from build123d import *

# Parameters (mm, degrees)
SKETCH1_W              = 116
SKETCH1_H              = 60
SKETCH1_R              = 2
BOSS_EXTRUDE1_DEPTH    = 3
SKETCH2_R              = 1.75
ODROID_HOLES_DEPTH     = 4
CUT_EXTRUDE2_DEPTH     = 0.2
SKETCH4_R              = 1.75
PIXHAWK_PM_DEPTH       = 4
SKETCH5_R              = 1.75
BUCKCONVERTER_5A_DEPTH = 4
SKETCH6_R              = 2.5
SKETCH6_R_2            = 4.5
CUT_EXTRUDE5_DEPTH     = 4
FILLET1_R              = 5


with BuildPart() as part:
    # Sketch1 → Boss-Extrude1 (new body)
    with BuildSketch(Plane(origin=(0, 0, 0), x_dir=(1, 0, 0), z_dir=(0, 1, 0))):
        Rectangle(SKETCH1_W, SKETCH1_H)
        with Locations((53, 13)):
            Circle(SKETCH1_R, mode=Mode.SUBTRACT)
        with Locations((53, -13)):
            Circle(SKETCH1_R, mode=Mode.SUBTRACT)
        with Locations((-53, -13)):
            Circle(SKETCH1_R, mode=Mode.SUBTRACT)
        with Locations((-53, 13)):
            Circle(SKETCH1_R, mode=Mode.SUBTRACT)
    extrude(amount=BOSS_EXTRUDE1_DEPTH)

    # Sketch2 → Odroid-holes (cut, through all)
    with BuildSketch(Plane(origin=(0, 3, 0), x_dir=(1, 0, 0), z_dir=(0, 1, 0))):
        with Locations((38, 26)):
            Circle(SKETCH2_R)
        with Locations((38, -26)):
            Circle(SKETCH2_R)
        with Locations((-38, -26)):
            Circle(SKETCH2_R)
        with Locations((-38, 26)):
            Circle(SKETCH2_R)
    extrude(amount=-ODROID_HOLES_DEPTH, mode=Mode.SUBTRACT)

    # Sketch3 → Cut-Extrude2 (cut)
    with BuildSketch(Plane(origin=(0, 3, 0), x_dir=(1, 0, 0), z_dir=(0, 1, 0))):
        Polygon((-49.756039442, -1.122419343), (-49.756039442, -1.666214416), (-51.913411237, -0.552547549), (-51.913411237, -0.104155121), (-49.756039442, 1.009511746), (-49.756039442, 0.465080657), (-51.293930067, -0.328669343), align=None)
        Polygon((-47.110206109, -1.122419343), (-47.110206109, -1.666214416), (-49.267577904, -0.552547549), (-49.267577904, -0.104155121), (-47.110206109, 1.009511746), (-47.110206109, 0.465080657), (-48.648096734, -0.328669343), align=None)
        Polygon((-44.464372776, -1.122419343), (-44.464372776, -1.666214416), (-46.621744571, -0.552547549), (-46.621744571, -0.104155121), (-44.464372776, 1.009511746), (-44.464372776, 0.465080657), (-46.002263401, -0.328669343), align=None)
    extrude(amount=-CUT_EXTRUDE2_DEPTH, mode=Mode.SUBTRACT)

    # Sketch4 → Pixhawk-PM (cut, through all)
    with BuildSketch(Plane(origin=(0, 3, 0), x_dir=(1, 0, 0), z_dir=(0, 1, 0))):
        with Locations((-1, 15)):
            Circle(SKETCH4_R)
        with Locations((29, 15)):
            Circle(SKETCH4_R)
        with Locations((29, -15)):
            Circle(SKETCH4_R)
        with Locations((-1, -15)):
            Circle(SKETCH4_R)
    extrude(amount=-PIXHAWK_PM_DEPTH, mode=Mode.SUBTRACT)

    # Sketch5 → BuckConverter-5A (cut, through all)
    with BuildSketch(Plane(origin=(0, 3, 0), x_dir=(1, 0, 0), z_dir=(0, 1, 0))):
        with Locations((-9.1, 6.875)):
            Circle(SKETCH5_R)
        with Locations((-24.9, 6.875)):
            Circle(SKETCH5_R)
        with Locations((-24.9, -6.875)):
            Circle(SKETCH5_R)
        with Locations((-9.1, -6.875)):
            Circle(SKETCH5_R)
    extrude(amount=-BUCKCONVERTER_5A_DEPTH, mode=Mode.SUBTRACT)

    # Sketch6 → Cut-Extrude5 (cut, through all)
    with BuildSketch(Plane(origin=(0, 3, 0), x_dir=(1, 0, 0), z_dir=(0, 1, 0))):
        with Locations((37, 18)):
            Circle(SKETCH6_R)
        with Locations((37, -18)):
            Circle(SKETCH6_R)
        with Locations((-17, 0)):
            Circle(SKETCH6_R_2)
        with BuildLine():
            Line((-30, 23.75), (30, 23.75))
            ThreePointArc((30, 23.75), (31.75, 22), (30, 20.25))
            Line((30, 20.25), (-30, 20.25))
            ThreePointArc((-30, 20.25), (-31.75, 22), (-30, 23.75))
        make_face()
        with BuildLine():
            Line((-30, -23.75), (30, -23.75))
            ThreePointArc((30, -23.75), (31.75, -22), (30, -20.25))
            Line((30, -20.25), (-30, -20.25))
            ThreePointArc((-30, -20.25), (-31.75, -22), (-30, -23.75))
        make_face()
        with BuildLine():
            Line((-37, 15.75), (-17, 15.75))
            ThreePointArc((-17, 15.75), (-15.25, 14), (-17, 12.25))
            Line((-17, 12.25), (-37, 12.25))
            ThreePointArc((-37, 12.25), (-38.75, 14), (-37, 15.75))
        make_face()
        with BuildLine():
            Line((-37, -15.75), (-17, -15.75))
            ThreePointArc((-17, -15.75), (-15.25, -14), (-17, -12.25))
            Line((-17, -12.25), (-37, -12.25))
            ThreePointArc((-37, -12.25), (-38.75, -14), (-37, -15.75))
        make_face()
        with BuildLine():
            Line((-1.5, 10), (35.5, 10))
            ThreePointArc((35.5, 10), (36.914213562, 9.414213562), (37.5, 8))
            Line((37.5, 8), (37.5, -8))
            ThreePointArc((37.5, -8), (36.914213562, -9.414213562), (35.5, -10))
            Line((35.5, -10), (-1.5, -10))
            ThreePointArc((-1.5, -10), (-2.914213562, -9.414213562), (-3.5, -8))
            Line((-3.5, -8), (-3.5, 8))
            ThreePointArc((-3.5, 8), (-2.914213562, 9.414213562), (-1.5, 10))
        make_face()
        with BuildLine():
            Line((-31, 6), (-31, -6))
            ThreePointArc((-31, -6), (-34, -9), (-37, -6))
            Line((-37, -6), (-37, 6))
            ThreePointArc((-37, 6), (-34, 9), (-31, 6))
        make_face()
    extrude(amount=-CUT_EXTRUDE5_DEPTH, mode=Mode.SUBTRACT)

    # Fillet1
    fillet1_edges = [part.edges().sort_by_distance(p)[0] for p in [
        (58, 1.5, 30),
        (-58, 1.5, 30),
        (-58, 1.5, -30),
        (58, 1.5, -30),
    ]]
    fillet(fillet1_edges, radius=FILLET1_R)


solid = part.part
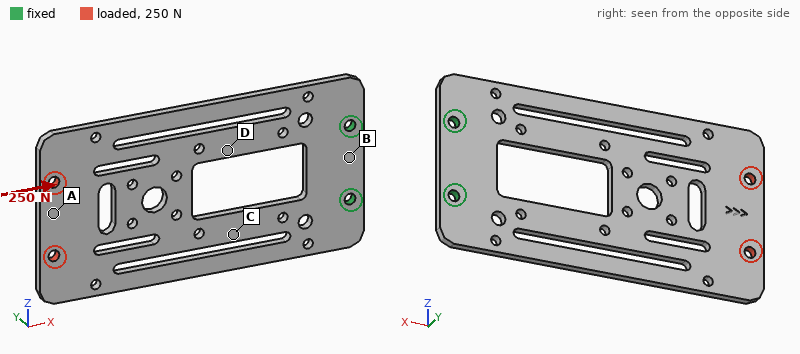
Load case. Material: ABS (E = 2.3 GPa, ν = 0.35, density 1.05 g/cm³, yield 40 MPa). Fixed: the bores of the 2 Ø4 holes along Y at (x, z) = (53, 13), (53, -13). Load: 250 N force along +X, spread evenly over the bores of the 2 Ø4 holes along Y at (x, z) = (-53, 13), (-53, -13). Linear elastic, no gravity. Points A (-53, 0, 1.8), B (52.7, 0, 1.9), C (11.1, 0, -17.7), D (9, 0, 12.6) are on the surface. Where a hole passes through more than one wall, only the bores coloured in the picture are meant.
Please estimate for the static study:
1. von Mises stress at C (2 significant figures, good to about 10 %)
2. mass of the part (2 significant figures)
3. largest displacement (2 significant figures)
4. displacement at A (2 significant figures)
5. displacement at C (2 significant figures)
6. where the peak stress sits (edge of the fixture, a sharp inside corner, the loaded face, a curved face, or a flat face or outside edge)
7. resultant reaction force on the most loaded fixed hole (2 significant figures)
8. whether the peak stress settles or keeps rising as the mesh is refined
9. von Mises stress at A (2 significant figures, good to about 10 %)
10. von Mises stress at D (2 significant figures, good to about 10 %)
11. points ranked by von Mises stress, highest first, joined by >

2.5 MPa
16 g
0.17 mm
0.16 mm
0.070 mm
a sharp inside corner
130 N
keeps rising
1.2 MPa
3.3 MPa
D > C > A > B
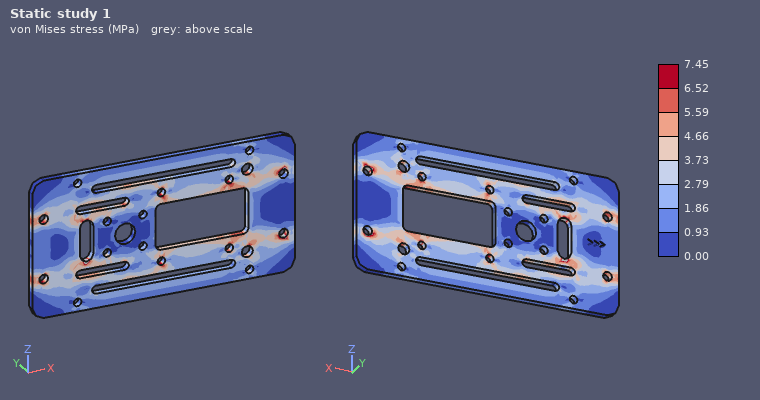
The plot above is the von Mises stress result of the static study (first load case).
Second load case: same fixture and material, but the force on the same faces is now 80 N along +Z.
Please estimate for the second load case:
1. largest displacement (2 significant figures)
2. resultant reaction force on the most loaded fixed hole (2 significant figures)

1.6 mm
280 N
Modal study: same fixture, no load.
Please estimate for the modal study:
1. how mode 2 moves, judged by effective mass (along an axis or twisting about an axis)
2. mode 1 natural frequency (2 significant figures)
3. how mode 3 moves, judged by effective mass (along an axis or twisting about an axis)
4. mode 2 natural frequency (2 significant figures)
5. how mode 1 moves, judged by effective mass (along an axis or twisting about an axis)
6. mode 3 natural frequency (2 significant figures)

twisting about X
49 Hz
along Y
180 Hz
along Y
340 Hz
